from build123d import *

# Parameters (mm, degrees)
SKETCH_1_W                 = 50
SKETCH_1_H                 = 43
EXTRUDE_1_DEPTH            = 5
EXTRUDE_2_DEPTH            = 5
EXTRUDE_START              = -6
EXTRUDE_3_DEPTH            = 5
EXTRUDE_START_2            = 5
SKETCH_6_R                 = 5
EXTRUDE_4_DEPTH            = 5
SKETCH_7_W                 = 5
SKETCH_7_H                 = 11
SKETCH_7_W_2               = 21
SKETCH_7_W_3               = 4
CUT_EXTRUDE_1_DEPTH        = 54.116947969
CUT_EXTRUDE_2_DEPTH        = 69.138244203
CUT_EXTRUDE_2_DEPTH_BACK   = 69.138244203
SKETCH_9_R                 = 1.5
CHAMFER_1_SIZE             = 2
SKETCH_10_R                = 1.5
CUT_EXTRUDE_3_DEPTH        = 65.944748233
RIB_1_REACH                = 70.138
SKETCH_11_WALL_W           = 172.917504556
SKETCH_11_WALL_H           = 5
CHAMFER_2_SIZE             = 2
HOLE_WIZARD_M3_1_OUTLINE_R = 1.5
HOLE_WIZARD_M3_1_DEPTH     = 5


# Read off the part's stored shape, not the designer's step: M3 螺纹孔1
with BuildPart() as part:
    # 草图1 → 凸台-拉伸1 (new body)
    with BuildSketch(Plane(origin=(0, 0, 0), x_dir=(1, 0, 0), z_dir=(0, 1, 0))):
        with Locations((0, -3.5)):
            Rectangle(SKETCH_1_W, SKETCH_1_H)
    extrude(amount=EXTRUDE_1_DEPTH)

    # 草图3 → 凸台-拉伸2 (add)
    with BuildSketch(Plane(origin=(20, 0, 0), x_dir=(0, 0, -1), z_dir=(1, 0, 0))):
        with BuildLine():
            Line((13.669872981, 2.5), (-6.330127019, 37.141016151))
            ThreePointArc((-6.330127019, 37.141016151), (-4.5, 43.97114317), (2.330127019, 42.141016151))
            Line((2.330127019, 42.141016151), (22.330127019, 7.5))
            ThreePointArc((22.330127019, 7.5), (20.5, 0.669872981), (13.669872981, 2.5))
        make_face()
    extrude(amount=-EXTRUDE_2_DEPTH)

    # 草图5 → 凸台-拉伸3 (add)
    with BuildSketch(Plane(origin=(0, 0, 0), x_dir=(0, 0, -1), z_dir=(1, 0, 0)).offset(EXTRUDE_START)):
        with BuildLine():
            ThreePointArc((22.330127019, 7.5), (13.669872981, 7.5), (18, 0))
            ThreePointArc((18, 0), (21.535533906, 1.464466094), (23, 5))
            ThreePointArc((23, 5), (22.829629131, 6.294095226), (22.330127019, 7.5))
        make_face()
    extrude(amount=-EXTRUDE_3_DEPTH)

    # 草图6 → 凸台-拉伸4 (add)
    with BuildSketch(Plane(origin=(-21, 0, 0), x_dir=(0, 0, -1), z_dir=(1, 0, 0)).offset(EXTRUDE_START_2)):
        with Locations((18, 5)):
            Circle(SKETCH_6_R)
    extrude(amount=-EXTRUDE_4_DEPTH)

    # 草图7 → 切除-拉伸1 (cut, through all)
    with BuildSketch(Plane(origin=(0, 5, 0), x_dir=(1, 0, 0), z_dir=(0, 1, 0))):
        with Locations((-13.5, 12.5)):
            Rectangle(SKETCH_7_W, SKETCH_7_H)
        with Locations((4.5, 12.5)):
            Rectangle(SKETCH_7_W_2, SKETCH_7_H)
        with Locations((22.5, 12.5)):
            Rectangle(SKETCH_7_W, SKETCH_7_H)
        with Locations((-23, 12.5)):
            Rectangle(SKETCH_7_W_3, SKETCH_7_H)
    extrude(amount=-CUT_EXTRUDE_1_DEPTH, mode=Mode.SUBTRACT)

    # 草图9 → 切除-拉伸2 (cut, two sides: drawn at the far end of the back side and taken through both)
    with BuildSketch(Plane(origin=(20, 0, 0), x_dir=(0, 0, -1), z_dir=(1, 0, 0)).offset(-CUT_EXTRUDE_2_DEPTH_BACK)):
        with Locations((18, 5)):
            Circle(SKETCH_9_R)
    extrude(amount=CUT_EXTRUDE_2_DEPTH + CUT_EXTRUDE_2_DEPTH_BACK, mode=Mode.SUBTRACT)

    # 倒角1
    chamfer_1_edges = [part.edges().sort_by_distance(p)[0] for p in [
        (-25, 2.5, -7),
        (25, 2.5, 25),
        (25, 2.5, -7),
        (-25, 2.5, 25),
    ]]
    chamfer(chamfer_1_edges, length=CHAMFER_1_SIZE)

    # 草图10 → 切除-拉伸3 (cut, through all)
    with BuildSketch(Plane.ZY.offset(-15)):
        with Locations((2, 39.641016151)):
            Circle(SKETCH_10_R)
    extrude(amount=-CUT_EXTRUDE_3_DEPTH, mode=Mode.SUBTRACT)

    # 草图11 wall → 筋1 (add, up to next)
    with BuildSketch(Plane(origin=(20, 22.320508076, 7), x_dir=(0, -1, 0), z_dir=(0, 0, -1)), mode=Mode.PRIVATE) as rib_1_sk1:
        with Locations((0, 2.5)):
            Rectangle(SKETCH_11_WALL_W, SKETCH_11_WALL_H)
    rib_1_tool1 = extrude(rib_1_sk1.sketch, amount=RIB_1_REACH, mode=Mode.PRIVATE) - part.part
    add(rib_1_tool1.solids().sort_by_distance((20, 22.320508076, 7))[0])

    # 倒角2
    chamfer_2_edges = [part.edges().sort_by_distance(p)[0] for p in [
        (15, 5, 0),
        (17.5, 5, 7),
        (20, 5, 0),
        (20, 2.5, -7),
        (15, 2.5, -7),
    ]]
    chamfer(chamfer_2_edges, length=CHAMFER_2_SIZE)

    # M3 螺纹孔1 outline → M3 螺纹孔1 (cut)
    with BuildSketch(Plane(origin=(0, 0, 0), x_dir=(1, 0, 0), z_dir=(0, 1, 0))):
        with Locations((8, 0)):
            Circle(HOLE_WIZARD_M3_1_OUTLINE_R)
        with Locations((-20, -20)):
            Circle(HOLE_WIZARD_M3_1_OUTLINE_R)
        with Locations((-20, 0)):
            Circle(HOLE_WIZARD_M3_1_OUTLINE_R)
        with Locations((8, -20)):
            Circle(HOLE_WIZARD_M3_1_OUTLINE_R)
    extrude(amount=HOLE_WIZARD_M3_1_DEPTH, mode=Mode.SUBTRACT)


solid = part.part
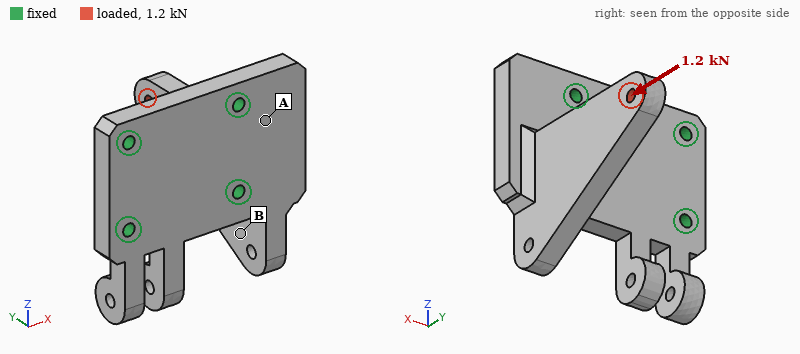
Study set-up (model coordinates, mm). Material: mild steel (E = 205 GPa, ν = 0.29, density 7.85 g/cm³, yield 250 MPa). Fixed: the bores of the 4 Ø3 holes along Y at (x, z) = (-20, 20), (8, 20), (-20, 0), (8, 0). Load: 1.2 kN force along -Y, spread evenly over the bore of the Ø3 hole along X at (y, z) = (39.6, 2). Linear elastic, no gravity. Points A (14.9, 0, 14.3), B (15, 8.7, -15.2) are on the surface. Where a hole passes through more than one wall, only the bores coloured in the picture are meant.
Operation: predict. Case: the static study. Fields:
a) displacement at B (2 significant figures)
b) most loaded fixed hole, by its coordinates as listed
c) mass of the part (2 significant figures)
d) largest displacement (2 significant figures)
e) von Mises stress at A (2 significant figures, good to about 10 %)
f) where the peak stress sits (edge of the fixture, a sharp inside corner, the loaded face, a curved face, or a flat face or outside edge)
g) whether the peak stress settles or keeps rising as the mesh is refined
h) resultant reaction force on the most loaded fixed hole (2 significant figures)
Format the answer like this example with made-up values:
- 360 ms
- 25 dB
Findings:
- 10 µm
- (8, 0)
- 100 g
- 51 µm
- 29 MPa
- edge of the fixture
- keeps rising
- 1.1 kN
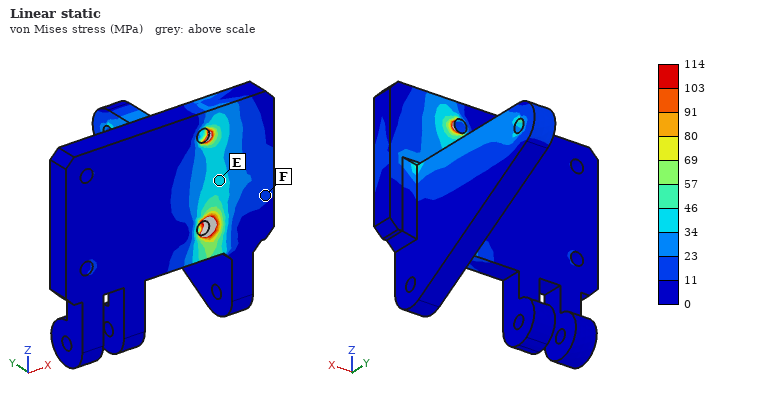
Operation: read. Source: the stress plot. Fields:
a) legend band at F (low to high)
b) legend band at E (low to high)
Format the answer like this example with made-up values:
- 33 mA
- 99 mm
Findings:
- 11 to 23 MPa
- 34 to 46 MPa
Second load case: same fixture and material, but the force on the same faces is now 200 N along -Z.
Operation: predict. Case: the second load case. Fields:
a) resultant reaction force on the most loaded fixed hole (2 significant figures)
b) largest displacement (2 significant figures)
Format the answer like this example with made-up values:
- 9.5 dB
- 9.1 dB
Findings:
- 320 N
- 30 µm
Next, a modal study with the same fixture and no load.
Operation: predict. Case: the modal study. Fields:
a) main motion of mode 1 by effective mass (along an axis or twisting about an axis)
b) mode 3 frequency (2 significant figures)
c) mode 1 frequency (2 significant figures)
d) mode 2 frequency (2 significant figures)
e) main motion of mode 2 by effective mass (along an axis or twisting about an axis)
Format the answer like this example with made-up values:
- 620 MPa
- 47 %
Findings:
- along X
- 7000 Hz
- 2500 Hz
- 4300 Hz
- along Z
